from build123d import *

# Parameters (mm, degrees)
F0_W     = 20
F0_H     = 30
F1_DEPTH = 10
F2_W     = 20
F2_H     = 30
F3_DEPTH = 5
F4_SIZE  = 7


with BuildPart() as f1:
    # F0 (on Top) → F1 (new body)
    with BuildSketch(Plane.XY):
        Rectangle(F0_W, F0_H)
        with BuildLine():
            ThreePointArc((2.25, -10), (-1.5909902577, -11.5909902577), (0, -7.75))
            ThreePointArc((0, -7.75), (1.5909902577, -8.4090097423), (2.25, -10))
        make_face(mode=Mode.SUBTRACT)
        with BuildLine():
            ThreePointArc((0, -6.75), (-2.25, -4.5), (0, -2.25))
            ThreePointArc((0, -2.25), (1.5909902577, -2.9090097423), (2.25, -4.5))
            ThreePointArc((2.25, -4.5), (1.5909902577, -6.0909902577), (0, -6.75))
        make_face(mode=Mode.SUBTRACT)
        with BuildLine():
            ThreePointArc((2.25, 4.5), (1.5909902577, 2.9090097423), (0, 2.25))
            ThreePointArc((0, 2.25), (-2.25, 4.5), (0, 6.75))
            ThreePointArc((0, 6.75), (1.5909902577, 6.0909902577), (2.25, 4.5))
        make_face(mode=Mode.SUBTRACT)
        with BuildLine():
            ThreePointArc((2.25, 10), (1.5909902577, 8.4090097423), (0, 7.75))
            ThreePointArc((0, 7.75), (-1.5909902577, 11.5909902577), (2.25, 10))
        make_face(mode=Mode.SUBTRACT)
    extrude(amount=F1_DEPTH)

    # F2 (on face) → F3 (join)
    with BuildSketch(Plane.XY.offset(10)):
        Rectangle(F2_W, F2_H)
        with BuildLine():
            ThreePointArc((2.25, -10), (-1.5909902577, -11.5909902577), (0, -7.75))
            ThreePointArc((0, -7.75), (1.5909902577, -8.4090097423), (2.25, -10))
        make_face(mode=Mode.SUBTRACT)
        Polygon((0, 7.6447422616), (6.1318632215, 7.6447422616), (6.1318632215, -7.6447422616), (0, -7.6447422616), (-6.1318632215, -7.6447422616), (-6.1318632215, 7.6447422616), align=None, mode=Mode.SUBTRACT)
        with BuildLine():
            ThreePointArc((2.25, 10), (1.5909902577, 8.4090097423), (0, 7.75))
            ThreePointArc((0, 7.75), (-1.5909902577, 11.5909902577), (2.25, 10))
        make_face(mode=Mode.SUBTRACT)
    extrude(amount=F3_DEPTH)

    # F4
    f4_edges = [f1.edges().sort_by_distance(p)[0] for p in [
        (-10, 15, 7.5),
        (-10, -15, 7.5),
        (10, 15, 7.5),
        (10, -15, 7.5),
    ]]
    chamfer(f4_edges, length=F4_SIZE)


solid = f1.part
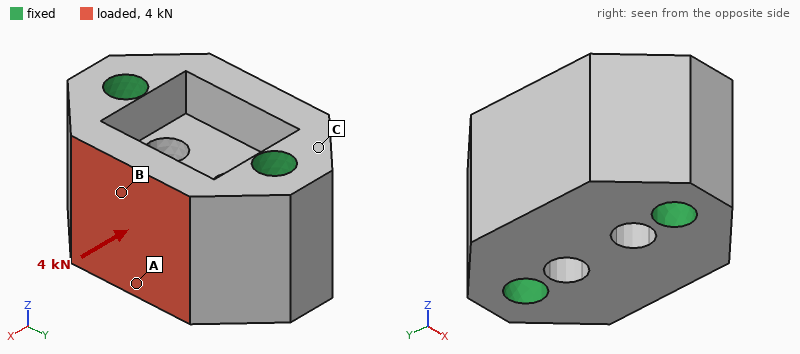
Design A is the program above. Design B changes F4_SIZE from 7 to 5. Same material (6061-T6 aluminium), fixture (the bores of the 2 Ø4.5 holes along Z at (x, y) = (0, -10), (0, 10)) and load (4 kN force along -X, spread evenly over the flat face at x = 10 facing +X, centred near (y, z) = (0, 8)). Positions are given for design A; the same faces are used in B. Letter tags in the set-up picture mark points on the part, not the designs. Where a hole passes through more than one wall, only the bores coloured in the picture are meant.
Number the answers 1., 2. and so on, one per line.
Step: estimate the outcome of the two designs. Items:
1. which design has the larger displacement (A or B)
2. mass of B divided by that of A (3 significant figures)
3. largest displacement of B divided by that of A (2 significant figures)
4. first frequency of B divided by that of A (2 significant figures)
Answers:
1. A
2. 1.12
3. 0.79
4. 1.0
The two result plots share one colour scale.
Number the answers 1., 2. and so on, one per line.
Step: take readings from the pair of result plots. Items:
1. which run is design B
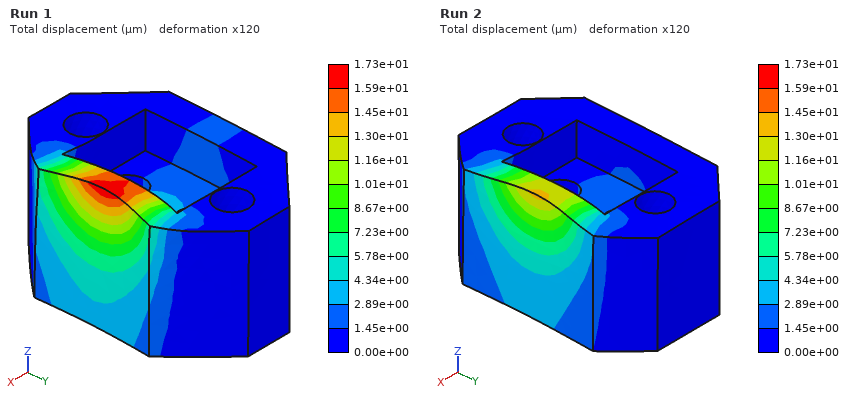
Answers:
1. Run 2
